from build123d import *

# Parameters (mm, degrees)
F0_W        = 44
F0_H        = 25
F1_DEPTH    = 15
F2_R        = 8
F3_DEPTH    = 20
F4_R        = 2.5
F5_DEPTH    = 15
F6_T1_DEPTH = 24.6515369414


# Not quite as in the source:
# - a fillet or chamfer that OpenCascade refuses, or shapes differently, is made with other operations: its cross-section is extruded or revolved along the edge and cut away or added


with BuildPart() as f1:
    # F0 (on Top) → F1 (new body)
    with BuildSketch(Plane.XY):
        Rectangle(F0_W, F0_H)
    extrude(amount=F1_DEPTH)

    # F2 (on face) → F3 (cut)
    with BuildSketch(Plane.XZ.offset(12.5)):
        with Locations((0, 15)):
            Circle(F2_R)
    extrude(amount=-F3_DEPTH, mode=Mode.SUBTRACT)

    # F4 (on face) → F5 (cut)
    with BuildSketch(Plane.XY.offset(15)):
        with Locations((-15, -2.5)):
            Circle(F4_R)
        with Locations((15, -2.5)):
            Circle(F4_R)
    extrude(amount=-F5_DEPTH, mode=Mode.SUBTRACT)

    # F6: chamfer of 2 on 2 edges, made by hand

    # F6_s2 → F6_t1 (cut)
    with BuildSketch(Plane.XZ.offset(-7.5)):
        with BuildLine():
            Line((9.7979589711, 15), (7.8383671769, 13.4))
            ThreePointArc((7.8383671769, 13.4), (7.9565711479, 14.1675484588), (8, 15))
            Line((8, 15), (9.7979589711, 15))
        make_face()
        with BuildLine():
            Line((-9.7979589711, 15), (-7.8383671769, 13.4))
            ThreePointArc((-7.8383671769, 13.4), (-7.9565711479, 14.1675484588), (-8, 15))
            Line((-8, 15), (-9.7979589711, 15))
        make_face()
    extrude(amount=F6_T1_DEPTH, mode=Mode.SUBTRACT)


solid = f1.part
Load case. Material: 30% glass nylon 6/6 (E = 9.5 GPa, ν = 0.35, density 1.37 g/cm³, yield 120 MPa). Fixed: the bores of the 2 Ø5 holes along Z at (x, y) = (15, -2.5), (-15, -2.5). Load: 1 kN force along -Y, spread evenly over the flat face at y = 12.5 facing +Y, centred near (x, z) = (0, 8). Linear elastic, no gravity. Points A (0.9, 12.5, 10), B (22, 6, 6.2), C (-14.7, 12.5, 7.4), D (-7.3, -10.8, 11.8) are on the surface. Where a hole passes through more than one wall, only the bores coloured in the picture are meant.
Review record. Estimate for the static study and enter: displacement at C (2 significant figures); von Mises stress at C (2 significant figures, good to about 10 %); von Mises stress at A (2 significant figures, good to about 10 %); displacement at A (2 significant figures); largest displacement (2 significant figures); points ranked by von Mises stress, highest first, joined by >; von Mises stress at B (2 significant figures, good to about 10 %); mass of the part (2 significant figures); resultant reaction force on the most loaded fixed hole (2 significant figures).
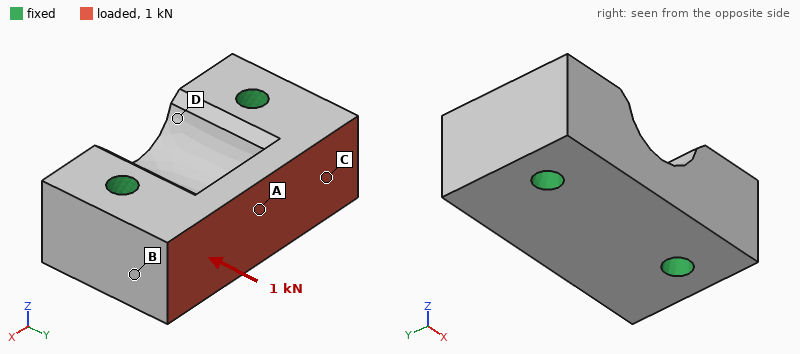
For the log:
2.9 µm
1.9 MPa
3.2 MPa
7.8 µm
12 µm
A > C > B > D
1.1 MPa
19 g
510 N
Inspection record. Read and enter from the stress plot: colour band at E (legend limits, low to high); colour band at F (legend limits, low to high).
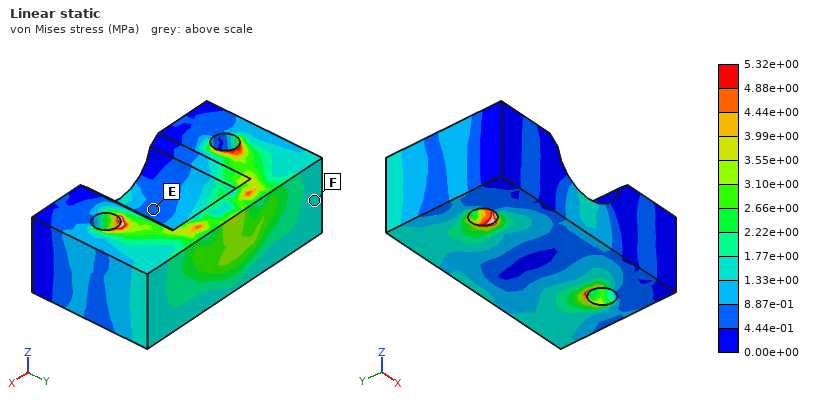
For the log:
4.44e-01 to 8.87e-01 MPa
1.33e+00 to 1.77e+00 MPa
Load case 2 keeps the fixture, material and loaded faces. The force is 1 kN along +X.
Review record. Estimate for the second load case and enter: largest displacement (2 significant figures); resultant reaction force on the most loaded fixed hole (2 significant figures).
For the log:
17 µm
630 N
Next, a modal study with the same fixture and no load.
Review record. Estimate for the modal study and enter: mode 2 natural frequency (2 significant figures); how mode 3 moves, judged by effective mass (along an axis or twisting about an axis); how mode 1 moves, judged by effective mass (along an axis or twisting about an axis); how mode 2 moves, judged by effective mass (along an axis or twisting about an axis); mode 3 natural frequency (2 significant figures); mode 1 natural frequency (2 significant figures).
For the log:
18 kHz
along Y
along Z
along X
21 kHz
15 kHz
